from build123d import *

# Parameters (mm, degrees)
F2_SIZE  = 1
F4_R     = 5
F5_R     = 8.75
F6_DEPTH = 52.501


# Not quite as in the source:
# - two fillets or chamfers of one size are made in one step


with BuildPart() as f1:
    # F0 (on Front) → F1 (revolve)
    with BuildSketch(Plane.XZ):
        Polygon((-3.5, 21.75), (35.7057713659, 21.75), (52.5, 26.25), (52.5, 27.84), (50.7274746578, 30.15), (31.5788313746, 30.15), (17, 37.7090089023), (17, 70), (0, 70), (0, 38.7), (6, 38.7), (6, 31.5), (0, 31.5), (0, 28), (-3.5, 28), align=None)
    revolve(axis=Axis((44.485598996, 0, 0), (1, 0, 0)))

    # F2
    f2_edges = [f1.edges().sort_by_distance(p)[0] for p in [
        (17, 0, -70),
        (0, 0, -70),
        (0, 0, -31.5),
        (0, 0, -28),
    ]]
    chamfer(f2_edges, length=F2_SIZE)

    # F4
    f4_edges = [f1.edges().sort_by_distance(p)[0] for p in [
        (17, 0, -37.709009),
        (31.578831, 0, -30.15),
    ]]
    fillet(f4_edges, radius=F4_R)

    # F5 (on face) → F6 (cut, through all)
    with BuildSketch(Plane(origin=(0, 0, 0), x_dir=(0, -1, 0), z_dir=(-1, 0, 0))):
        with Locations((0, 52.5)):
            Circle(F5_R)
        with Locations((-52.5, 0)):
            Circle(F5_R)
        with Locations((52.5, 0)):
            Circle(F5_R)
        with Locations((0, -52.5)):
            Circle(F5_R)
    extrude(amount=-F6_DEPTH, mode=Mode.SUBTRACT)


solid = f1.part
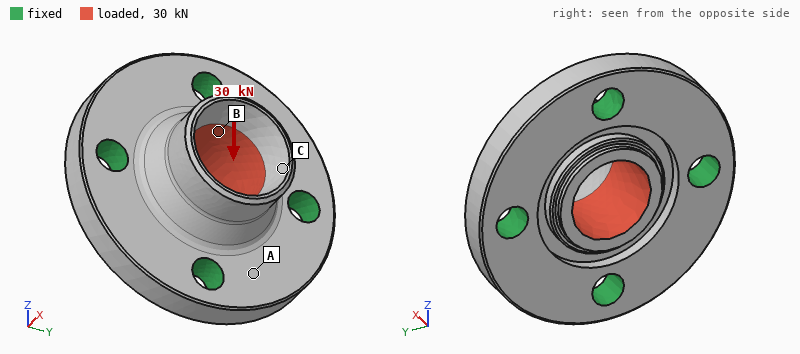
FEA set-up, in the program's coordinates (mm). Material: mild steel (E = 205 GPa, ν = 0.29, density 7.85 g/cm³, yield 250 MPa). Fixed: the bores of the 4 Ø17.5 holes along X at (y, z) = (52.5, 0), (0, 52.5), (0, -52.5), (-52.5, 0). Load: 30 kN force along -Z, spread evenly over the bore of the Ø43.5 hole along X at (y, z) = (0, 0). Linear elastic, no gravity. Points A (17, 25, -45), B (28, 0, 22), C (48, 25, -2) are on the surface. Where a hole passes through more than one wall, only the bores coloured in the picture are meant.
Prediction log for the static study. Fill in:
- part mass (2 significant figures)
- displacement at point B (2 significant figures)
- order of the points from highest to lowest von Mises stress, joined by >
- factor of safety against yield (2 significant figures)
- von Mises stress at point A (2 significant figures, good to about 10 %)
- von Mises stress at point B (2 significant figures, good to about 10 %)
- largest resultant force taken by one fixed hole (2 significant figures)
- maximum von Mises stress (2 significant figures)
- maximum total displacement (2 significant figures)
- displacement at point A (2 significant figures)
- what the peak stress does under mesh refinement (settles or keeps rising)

2.1 kg
3.1 µm
B > A > C
5.6
6.2 MPa
11 MPa
9.2 kN
44 MPa
3.5 µm
1.3 µm
settles
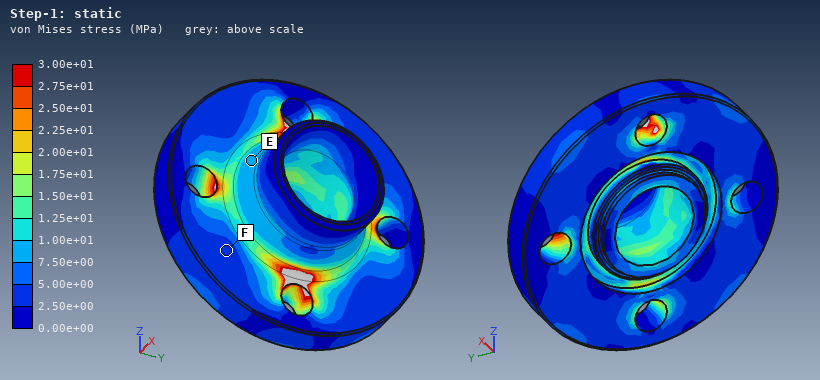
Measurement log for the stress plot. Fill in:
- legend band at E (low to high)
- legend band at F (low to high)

7.50e+00 to 1.00e+01 MPa
2.50e+00 to 5.00e+00 MPa
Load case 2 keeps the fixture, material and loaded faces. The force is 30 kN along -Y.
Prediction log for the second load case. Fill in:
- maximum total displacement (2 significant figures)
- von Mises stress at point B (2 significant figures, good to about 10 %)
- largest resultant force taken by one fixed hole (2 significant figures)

3.5 µm
13 MPa
9.2 kN
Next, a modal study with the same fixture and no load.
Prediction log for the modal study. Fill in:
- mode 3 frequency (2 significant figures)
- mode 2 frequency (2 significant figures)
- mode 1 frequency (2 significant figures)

11 kHz
11 kHz
11 kHz
